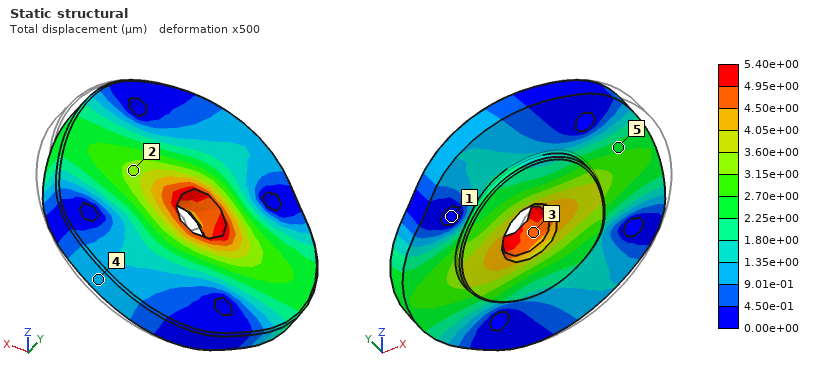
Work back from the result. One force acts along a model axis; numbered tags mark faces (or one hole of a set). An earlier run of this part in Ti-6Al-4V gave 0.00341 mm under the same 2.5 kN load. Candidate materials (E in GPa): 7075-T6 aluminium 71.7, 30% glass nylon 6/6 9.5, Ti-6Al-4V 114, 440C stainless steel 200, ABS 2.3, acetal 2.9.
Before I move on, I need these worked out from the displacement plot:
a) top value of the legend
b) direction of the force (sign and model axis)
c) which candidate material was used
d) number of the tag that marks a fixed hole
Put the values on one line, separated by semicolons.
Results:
5.40e+00 µm; -X; 7075-T6 aluminium; 1
